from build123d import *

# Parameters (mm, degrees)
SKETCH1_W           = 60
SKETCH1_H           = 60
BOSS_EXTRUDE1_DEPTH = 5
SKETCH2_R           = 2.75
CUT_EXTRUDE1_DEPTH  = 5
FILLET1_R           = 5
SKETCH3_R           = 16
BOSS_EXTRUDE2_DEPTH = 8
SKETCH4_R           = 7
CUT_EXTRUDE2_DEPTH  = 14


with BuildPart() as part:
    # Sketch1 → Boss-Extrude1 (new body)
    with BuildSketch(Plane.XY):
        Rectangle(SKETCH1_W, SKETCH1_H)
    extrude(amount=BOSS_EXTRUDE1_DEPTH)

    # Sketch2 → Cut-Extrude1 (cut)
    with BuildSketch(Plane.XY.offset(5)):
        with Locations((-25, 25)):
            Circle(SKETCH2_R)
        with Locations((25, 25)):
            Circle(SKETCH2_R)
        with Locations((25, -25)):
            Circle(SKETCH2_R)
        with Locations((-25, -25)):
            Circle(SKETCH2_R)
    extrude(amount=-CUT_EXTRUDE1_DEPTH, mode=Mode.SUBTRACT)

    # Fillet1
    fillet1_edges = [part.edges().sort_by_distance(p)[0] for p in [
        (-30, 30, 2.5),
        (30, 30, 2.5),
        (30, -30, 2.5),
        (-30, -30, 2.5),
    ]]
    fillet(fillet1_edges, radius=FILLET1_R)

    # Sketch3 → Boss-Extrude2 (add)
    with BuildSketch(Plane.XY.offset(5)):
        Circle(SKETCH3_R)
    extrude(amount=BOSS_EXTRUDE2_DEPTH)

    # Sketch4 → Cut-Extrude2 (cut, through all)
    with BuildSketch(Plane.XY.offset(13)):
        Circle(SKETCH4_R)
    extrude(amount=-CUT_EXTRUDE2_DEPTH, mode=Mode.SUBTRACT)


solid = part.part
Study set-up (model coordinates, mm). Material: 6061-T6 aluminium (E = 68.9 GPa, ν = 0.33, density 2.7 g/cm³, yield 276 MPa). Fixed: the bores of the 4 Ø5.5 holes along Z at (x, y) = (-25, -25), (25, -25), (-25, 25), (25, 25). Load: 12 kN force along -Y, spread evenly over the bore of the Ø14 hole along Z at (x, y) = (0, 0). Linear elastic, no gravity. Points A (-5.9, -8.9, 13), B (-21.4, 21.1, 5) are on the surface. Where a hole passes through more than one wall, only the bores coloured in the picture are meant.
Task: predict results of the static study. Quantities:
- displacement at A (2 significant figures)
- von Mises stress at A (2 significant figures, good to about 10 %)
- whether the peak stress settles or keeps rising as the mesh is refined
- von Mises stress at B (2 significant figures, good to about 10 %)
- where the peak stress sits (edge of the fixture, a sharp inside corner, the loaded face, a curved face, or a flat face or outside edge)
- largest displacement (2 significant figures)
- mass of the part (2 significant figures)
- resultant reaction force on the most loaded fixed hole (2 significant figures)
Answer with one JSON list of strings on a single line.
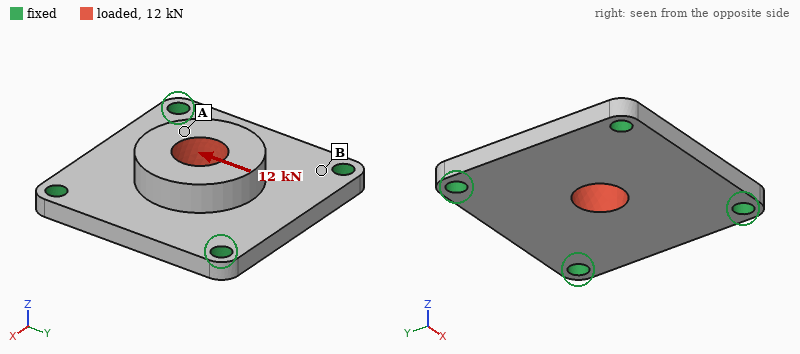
["39 µm", "19 MPa", "keeps rising", "55 MPa", "edge of the fixture", "45 µm", "59 g", "3.4 kN"]
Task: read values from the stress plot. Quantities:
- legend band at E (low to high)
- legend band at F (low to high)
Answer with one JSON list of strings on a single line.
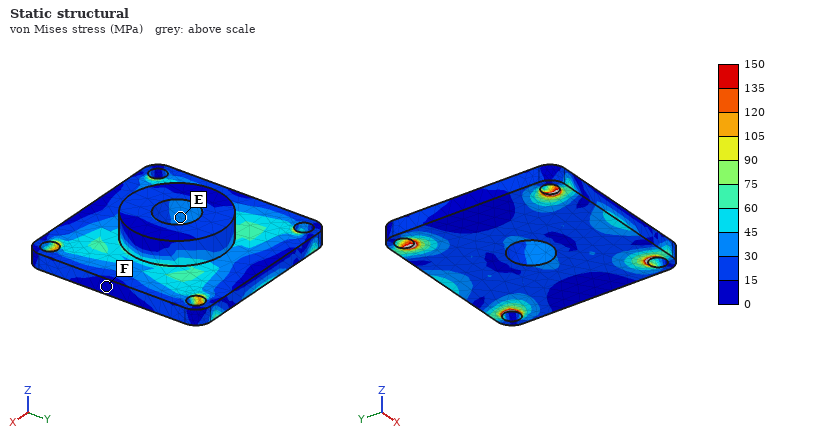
["30 to 45 MPa", "0 to 15 MPa"]
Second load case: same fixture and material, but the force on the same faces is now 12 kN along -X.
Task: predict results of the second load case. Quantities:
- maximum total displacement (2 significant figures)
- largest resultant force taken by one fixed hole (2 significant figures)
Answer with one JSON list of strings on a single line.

["45 µm", "3.4 kN"]
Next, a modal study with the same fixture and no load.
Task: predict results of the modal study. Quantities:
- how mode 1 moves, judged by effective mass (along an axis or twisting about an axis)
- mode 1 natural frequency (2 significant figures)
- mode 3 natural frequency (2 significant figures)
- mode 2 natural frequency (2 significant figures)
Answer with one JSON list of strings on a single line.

["along Z", "7000 Hz", "11 kHz", "11 kHz"]
